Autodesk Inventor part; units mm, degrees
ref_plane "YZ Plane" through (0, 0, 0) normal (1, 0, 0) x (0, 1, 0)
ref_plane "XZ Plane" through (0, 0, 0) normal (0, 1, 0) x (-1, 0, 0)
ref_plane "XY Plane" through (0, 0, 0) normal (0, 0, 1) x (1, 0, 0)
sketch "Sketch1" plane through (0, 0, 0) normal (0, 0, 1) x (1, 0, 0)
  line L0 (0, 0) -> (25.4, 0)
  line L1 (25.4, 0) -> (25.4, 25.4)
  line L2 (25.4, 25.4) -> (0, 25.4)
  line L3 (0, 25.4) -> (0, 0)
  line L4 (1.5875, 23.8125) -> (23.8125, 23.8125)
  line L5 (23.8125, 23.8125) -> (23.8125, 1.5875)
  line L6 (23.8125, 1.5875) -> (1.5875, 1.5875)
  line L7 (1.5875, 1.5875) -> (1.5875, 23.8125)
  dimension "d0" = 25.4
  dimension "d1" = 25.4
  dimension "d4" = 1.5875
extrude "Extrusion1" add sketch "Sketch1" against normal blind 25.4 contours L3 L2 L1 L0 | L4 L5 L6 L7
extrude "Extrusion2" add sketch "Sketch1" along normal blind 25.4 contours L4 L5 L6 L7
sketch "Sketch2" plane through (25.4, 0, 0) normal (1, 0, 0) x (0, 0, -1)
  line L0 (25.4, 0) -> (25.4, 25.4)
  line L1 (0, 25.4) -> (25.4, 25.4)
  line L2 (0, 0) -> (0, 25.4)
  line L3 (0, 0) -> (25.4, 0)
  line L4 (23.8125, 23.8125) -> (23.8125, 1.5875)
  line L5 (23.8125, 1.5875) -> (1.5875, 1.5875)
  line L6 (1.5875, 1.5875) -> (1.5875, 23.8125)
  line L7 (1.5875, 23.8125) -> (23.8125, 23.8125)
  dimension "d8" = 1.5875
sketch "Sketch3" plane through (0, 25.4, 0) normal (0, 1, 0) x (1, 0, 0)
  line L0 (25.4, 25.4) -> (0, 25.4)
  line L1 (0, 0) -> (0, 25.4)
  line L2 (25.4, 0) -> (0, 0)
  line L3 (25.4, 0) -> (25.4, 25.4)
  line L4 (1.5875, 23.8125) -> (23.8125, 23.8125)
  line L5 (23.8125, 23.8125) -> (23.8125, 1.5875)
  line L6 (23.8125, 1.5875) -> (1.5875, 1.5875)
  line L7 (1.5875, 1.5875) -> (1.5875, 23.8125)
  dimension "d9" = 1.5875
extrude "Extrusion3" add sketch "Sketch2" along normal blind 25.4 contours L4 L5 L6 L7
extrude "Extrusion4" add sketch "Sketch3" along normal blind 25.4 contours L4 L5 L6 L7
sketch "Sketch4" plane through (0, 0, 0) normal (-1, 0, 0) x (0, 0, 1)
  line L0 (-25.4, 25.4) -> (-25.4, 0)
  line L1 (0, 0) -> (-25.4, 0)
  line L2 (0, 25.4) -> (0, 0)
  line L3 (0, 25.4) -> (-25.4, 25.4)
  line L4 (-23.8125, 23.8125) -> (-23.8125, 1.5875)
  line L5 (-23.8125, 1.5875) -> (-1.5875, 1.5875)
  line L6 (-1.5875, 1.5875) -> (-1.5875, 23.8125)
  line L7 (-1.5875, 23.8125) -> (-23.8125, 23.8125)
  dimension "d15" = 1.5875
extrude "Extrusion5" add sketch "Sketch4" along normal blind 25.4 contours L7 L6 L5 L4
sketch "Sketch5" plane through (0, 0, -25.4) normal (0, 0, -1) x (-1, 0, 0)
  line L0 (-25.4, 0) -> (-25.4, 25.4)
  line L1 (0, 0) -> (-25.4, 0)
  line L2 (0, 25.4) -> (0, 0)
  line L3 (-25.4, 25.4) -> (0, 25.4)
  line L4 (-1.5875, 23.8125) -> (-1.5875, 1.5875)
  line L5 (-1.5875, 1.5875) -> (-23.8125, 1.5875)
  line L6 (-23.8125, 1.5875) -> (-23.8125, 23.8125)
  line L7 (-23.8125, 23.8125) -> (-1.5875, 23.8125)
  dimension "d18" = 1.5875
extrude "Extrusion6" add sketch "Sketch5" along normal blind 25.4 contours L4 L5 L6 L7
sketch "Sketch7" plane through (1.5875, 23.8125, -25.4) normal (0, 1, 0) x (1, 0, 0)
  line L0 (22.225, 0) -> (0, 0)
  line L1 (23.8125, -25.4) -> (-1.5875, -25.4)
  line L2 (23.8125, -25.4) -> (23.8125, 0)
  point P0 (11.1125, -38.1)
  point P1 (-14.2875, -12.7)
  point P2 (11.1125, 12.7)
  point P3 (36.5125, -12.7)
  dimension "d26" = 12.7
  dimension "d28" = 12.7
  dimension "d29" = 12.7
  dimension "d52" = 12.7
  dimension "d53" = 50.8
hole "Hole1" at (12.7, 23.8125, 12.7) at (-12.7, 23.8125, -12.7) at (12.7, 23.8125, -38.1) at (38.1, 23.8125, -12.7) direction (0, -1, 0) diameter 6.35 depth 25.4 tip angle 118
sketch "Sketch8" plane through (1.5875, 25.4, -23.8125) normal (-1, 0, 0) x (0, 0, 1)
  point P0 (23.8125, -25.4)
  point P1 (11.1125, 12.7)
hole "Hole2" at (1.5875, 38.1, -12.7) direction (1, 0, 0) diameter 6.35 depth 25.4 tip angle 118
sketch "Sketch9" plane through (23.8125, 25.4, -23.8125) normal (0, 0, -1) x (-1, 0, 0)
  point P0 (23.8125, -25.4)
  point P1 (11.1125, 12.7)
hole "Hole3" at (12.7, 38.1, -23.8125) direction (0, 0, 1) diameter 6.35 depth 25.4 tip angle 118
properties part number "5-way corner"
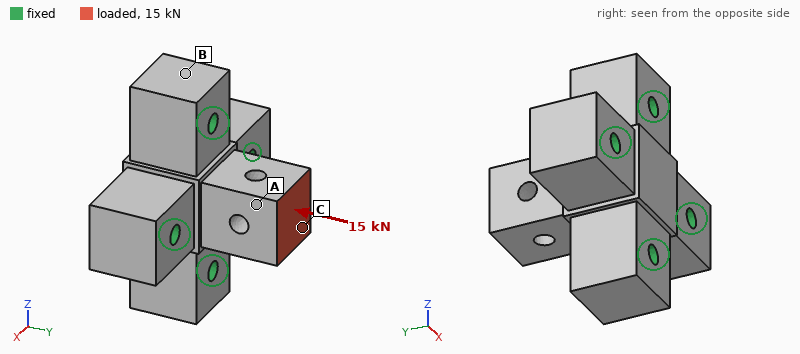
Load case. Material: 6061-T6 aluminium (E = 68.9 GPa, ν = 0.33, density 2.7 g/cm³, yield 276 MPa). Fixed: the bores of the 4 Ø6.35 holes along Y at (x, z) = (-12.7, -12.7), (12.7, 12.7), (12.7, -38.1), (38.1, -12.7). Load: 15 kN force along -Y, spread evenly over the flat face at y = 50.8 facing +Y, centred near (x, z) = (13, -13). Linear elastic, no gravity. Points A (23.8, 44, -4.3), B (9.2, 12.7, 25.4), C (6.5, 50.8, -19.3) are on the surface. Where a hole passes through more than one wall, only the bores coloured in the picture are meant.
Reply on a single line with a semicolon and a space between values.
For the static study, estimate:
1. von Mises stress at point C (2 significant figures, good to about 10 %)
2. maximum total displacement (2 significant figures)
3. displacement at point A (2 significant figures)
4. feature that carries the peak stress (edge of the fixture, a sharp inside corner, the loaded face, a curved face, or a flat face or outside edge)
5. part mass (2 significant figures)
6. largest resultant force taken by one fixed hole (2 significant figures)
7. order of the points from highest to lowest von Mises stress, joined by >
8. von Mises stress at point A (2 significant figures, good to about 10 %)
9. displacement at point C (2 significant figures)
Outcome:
26 MPa; 25 µm; 19 µm; a curved face; 200 g; 3.9 kN; A > C > B; 38 MPa; 23 µm
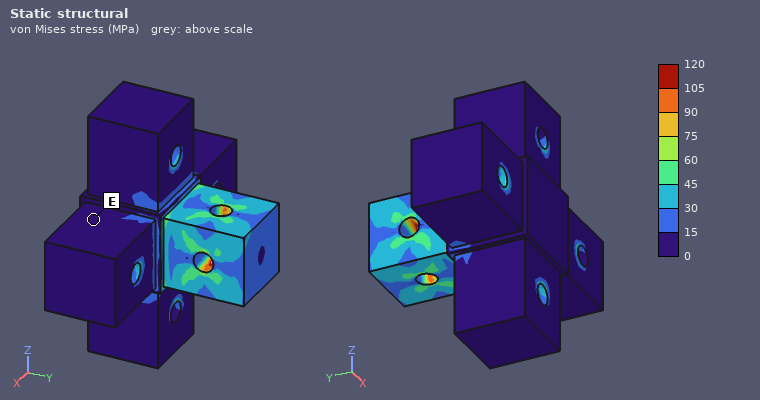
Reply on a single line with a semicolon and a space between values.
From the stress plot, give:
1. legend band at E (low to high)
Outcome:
0 to 15 MPa
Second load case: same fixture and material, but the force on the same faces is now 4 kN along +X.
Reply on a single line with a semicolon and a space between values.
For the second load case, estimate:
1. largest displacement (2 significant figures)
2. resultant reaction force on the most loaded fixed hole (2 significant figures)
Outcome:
55 µm; 3.5 kN
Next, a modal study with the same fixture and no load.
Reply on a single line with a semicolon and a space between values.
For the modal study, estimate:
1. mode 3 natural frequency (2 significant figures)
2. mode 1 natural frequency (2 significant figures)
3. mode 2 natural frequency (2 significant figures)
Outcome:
23 kHz; 13 kHz; 13 kHz
